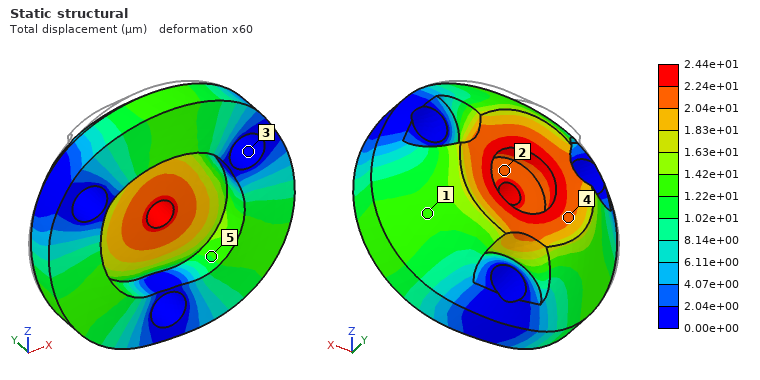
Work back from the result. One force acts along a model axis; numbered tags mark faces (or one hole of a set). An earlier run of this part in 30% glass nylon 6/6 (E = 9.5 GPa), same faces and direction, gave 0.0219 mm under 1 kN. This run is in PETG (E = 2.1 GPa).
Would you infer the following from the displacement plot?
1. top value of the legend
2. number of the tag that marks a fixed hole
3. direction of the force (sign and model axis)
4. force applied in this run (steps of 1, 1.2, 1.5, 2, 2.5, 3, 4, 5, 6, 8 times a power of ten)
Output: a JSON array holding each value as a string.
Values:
["2.44e+01 µm", "3", "-Y", "250 N"]
